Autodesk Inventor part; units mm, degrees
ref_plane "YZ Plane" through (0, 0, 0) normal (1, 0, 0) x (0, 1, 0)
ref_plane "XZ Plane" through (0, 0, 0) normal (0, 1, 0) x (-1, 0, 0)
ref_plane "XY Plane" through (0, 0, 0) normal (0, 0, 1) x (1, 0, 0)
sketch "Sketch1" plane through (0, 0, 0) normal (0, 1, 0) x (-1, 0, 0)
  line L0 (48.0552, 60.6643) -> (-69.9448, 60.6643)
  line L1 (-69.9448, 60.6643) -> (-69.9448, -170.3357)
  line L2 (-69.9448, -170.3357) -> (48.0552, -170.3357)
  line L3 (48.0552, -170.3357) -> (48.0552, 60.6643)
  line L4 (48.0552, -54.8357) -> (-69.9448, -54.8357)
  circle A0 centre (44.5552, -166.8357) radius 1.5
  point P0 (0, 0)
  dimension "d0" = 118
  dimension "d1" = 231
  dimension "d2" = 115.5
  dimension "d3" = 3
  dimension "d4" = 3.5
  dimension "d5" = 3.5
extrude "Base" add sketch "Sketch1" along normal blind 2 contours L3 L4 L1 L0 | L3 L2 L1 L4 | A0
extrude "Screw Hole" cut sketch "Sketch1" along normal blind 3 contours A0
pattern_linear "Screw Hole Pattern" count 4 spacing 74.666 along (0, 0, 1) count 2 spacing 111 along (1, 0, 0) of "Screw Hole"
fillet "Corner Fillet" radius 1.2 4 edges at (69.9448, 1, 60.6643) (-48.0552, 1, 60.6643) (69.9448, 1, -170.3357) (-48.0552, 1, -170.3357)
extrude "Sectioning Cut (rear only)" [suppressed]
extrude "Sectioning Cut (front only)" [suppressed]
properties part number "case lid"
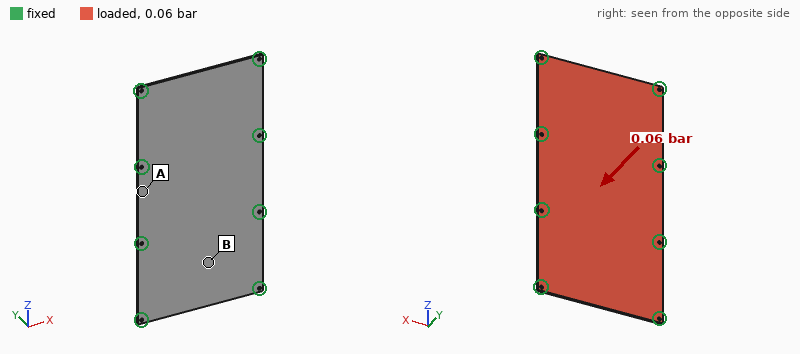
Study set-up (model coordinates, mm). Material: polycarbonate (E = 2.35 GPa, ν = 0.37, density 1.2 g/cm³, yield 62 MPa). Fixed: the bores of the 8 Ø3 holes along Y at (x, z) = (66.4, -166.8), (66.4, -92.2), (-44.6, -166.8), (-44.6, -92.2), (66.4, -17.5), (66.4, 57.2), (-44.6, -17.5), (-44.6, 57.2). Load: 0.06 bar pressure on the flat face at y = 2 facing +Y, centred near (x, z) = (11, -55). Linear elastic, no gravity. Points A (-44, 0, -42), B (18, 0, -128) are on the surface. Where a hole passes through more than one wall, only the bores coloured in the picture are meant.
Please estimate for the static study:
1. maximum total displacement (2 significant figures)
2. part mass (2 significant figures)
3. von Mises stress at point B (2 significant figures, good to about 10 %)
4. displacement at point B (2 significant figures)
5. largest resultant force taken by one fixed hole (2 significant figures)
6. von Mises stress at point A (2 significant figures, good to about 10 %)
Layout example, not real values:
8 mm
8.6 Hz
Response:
2.6 mm
65 g
5.3 MPa
2.6 mm
27 N
1.7 MPa
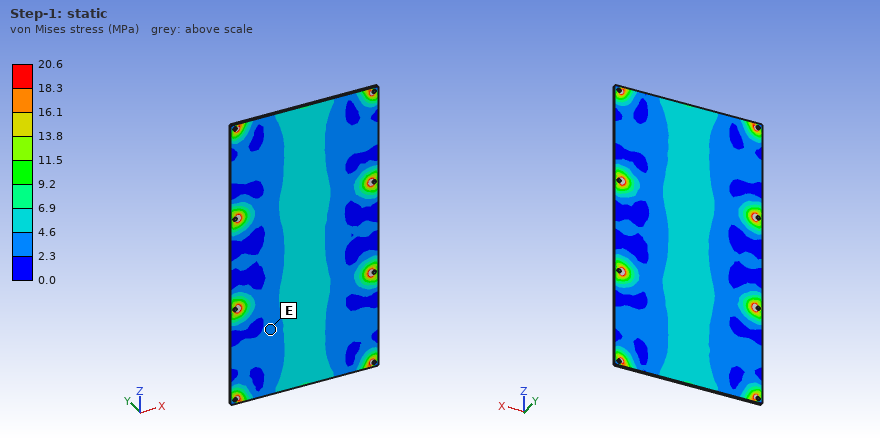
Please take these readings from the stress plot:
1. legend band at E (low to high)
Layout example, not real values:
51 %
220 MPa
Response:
2.3 to 4.6 MPa
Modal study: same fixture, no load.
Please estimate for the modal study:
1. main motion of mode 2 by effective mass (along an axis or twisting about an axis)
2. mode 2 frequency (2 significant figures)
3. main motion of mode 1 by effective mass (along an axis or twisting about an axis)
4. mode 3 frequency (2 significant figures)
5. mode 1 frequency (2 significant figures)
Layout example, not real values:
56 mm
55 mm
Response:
twisting about X
190 Hz
along Y
240 Hz
180 Hz
